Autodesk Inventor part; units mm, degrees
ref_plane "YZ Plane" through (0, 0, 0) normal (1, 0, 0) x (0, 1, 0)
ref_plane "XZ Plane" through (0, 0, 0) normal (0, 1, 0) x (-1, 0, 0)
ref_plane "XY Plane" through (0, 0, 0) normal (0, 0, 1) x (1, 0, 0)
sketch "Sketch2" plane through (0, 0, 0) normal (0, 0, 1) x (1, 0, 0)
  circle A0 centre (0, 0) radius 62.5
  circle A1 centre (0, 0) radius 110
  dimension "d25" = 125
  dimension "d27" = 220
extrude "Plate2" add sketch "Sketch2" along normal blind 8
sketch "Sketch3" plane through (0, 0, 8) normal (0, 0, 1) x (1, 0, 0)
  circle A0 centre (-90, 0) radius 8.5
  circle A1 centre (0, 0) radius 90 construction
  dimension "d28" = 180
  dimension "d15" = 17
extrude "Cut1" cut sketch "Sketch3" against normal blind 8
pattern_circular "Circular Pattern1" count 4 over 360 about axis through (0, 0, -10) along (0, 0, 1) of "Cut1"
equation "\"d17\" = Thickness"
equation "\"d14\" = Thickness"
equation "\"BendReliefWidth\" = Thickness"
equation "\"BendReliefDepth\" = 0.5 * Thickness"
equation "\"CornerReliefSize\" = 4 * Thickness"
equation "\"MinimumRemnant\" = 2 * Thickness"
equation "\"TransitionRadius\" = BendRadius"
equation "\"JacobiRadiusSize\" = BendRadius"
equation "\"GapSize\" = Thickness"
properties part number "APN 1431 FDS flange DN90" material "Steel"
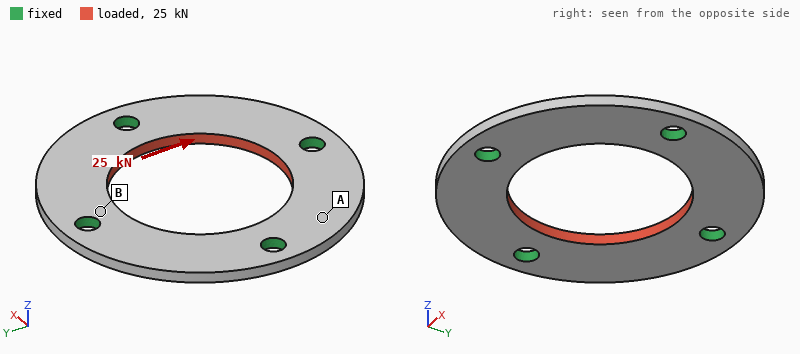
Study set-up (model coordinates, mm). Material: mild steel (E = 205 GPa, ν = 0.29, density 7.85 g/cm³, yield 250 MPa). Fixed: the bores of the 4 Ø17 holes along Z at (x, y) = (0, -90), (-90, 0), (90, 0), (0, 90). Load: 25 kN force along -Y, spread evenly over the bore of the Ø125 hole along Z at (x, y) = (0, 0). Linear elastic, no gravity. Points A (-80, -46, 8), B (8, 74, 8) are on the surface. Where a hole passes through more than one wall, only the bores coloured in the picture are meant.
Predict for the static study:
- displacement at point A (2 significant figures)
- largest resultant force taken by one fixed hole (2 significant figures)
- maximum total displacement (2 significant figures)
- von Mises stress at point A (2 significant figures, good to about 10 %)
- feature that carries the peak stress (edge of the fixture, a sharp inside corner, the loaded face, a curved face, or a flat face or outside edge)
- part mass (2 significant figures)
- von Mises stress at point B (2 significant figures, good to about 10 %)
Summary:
3.3 µm
7.1 kN
5.3 µm
7.8 MPa
edge of the fixture
1.6 kg
18 MPa
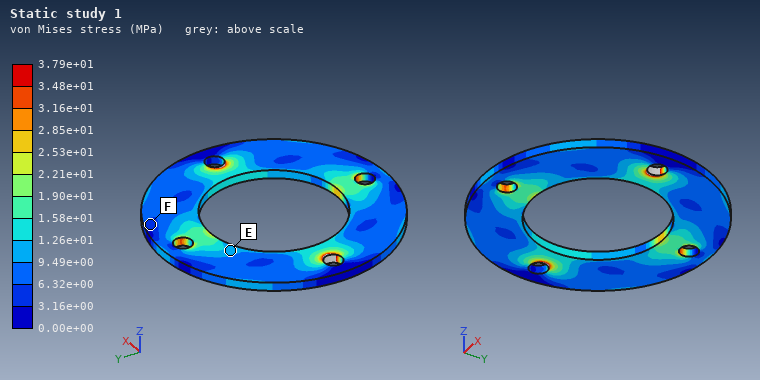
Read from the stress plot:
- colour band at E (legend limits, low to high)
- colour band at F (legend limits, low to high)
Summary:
9.49e+00 to 1.26e+01 MPa
3.16e+00 to 6.32e+00 MPa
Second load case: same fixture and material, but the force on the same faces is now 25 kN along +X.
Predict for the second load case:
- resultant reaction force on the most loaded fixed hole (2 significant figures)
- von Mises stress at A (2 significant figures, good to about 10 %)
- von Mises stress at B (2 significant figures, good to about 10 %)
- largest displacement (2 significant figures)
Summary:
7.1 kN
6.8 MPa
17 MPa
5.3 µm
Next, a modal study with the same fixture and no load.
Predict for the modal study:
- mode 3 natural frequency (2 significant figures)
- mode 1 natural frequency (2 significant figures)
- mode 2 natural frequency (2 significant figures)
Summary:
2200 Hz
2200 Hz
2200 Hz
